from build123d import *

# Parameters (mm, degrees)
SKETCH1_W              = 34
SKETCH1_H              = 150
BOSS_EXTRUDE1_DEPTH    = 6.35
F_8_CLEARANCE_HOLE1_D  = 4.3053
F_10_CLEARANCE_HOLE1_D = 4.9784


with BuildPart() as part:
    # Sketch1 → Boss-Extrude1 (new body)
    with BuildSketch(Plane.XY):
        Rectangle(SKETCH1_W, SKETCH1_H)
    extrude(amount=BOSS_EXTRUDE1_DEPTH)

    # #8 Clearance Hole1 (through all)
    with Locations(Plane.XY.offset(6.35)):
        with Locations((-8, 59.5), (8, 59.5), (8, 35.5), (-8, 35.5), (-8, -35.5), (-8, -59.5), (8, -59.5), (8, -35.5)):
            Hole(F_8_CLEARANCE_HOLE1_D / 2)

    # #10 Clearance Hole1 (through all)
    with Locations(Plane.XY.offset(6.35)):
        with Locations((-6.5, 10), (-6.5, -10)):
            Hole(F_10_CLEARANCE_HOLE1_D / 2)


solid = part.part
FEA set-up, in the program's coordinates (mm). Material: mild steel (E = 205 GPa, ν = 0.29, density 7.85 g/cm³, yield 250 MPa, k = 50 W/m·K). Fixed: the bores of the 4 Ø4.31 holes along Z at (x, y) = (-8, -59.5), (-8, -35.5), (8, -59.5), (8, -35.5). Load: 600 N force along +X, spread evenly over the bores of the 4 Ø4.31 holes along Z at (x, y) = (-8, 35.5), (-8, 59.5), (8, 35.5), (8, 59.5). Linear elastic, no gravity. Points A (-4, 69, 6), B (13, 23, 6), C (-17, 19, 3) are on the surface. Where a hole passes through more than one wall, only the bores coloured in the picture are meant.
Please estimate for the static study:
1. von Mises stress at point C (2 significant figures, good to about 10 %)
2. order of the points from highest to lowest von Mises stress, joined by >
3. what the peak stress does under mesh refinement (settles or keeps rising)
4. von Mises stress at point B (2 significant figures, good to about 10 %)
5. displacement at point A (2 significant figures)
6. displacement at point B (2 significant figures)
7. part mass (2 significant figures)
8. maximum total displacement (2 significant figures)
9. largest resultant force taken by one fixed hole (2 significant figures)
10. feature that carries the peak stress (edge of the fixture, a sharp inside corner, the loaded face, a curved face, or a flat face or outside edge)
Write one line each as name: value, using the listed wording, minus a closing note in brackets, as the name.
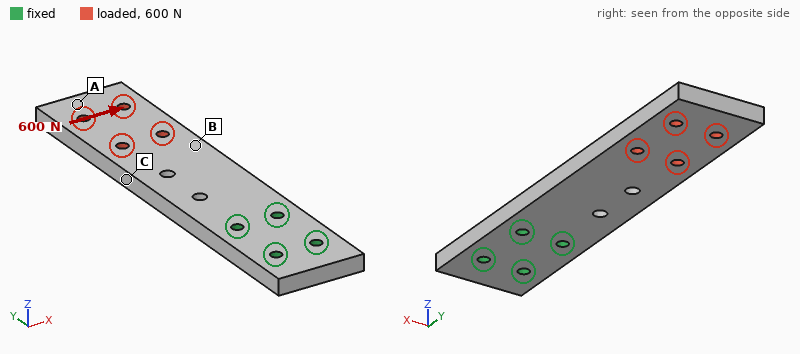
von Mises stress at point C: 15 MPa
order of the points from highest to lowest von Mises stress, joined by >: C > B > A
what the peak stress does under mesh refinement: keeps rising
von Mises stress at point B: 9.2 MPa
displacement at point A: 47 µm
displacement at point B: 22 µm
part mass: 250 g
maximum total displacement: 51 µm
largest resultant force taken by one fixed hole: 2.1 kN
feature that carries the peak stress: edge of the fixture
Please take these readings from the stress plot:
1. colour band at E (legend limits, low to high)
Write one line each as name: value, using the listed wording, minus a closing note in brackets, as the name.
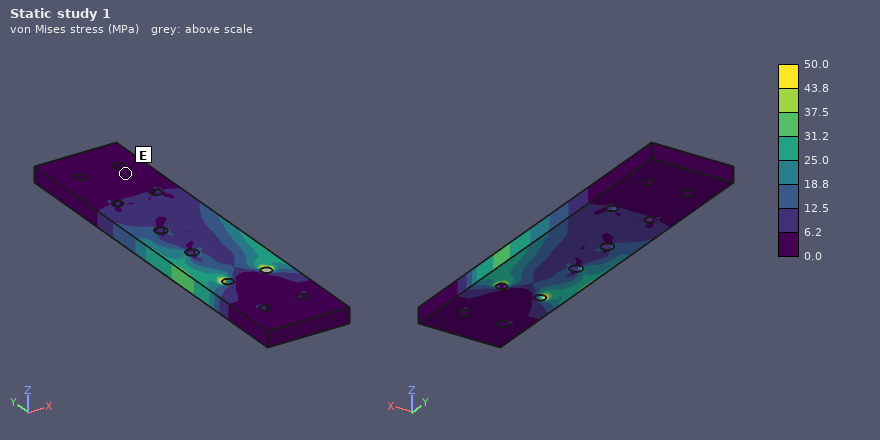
colour band at E: 0.0 to 6.2 MPa
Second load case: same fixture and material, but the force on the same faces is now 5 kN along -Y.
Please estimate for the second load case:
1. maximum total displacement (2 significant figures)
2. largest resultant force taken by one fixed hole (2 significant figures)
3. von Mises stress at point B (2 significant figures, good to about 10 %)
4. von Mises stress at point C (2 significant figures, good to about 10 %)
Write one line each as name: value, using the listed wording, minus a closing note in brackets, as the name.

maximum total displacement: 11 µm
largest resultant force taken by one fixed hole: 2.3 kN
von Mises stress at point B: 23 MPa
von Mises stress at point C: 27 MPa
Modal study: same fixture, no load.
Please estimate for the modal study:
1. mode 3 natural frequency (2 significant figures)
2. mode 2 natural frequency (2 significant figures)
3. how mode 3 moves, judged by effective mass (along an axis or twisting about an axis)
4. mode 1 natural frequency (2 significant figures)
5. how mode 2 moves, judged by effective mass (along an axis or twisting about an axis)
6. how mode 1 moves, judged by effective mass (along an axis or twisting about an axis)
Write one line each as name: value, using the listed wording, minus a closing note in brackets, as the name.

mode 3 natural frequency: 2600 Hz
mode 2 natural frequency: 2000 Hz
how mode 3 moves, judged by effective mass: twisting about Y
mode 1 natural frequency: 430 Hz
how mode 2 moves, judged by effective mass: along X
how mode 1 moves, judged by effective mass: along Z
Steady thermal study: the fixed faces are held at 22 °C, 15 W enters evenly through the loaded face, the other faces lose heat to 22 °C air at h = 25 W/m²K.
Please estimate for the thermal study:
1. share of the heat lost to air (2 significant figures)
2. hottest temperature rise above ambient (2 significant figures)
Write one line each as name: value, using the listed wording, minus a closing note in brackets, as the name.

share of the heat lost to air: 56 %
hottest temperature rise above ambient: 64 K
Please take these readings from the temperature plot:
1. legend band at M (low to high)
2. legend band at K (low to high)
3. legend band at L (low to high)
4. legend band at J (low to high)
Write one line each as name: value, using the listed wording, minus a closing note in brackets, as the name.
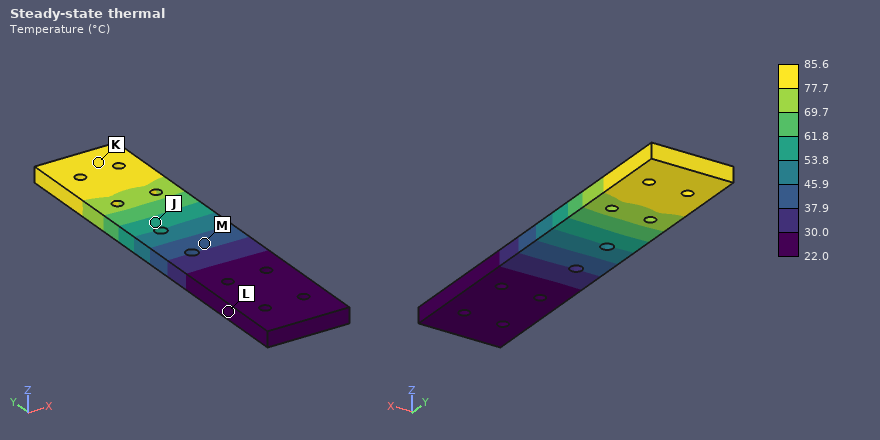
legend band at M: 37.9 to 45.9 °C
legend band at K: 77.7 to 85.6 °C
legend band at L: 22.0 to 30.0 °C
legend band at J: 53.8 to 61.8 °C
